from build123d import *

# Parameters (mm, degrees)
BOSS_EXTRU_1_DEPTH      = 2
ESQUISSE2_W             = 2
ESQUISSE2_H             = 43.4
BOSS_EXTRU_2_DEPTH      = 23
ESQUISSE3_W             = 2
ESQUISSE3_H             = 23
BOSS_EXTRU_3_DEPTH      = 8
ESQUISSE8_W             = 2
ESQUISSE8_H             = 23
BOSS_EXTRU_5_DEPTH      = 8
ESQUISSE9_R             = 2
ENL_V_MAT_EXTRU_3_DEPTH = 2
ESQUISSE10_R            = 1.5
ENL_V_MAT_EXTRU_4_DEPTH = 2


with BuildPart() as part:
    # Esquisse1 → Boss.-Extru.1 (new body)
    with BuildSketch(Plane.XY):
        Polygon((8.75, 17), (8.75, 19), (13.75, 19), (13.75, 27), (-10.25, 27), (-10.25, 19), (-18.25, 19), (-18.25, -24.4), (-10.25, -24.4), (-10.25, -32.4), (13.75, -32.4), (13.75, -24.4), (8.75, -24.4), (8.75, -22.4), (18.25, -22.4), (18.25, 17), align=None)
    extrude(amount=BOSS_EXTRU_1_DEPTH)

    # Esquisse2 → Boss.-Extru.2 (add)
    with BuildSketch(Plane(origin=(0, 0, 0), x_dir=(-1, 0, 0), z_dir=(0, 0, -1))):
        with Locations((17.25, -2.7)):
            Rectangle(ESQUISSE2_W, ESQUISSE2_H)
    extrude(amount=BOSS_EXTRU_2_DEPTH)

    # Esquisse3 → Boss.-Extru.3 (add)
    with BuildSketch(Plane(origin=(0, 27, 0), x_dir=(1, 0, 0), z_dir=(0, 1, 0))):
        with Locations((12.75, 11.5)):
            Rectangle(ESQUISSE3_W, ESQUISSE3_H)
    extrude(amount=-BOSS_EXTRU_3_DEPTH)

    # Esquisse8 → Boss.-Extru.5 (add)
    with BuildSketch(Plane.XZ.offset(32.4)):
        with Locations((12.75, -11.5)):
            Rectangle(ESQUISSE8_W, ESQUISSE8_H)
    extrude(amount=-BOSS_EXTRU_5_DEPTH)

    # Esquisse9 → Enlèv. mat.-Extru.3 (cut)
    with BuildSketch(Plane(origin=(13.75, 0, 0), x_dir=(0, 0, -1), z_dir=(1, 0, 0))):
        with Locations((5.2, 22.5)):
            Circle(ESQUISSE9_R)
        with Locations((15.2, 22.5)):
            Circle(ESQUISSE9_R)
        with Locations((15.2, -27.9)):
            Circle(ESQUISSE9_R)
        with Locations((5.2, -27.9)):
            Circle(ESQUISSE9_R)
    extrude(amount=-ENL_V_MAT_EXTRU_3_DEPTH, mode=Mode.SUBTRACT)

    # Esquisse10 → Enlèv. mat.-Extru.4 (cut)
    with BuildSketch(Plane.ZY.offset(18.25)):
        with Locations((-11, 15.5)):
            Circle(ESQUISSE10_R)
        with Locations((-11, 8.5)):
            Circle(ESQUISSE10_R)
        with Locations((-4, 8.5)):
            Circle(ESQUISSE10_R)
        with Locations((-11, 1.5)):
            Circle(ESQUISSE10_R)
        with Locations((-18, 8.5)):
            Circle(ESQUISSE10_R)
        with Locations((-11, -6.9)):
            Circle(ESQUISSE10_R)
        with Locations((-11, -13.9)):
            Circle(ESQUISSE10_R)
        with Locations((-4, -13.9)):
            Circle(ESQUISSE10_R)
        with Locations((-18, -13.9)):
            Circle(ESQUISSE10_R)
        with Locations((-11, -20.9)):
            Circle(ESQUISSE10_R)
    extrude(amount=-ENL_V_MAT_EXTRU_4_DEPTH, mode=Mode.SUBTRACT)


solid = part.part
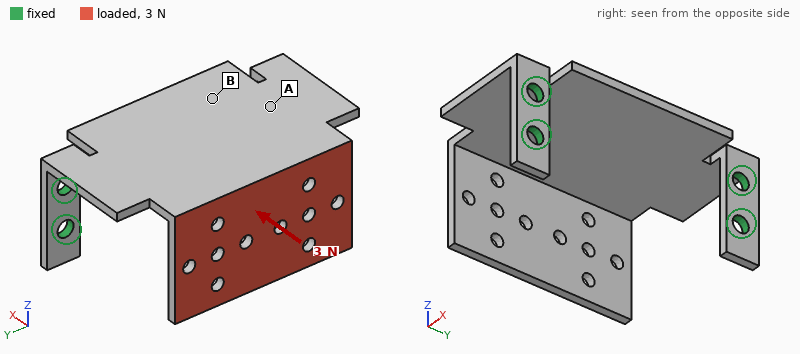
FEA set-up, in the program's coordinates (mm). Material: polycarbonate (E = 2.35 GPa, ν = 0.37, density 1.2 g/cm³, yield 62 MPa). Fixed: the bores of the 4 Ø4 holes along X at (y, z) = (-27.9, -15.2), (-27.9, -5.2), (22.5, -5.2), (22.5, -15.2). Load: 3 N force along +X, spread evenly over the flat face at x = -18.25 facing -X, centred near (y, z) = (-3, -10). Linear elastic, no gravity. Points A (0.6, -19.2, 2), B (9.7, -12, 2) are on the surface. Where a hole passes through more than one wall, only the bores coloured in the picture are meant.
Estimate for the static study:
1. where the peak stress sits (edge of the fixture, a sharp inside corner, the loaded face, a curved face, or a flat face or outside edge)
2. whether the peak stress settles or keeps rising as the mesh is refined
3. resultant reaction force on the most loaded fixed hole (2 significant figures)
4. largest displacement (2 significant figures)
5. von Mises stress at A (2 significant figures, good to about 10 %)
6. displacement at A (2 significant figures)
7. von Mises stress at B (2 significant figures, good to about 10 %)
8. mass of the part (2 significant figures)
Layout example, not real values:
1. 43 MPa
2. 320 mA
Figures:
1. a sharp inside corner
2. keeps rising
3. 1.6 N
4. 0.83 mm
5. 0.84 MPa
6. 0.14 mm
7. 0.30 MPa
8. 7.6 g
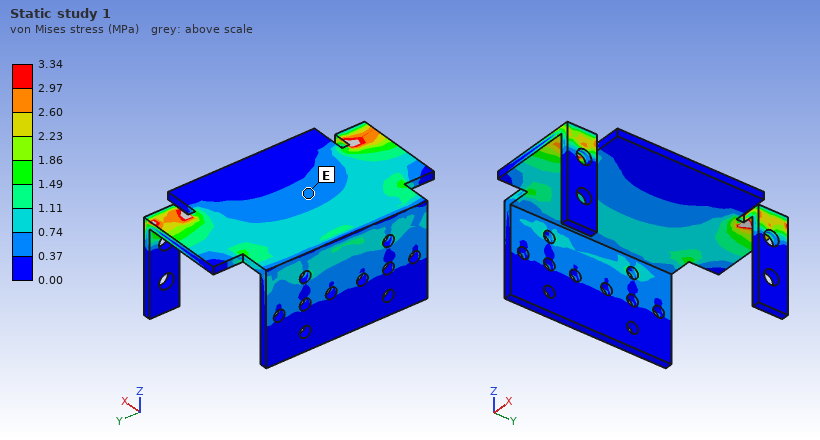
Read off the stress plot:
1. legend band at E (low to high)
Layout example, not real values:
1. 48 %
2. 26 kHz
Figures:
1. 0.37 to 0.74 MPa
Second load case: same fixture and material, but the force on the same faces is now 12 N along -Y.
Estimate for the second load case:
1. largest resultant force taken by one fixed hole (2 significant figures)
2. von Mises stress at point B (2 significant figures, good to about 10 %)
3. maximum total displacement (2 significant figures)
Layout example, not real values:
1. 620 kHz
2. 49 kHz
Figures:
1. 10 N
2. 1.5 MPa
3. 0.77 mm
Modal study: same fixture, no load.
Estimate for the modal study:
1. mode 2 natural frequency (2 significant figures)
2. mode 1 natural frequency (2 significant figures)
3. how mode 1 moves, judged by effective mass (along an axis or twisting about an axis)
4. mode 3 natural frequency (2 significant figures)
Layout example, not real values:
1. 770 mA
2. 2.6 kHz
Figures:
1. 380 Hz
2. 130 Hz
3. along Z
4. 500 Hz
